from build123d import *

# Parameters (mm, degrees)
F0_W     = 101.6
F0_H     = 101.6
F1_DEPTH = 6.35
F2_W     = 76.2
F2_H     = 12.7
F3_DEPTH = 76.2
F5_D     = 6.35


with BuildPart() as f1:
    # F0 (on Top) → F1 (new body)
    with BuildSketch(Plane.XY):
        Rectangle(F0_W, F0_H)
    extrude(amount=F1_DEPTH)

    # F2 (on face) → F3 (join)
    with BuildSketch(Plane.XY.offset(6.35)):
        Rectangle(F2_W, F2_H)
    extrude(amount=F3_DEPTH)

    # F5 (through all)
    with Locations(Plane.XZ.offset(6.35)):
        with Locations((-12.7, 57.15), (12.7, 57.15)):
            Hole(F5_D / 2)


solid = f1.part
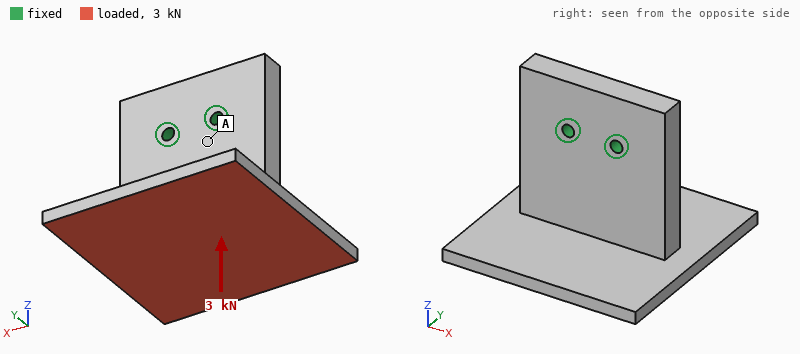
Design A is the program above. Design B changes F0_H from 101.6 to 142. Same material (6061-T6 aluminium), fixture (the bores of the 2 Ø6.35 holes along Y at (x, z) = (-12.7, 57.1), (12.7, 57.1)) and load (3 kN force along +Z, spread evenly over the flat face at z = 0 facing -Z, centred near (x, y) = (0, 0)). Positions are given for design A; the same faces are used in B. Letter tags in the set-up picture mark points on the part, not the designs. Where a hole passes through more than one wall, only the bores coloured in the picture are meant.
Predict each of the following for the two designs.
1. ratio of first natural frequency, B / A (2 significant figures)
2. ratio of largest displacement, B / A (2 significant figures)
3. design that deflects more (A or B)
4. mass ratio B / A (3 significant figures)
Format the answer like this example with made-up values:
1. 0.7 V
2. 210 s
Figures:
1. 0.67
2. 2.9
3. B
4. 1.19
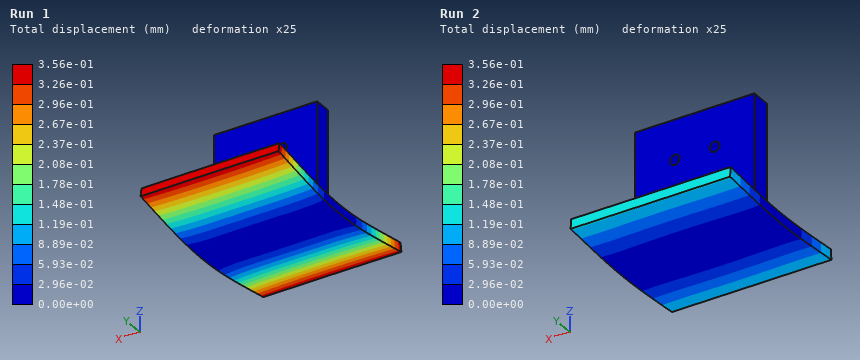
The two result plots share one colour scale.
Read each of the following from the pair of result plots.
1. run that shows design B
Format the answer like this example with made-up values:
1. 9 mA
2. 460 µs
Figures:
1. Run 1
